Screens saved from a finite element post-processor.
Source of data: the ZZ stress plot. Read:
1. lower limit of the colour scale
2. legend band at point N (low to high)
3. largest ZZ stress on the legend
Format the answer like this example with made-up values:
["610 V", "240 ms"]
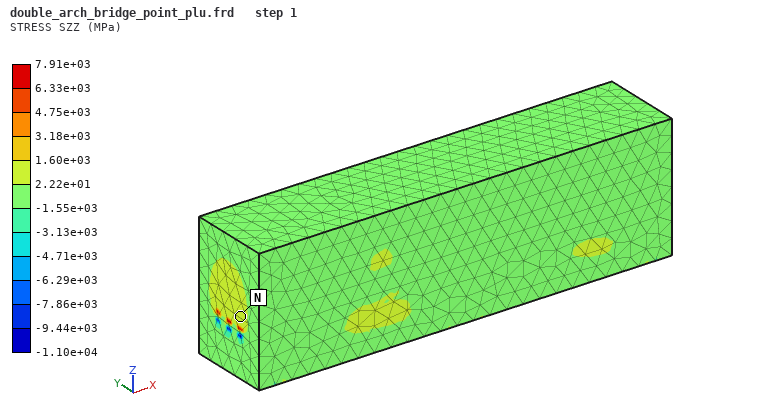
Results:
["-1.10e+04 MPa", "2.22e+01 to 1.60e+03 MPa", "7.91e+03 MPa"]
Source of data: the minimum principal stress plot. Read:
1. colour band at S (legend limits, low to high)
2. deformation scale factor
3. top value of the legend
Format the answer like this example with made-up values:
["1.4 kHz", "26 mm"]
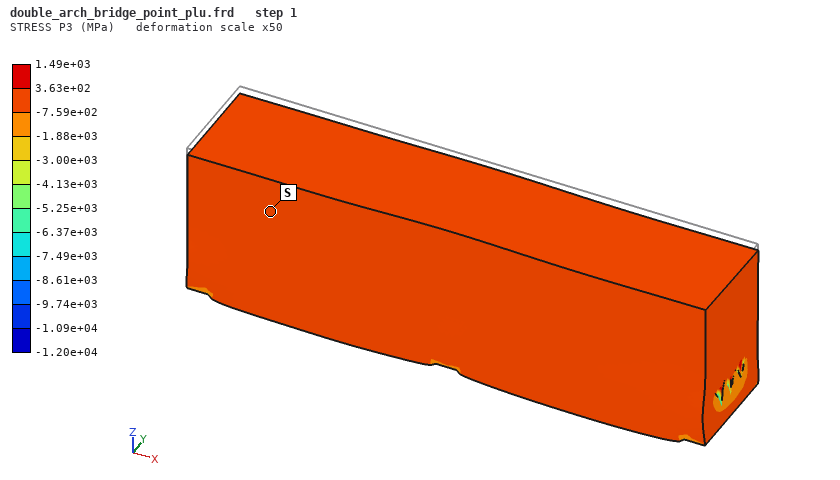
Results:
["-7.59e+02 to 3.63e+02 MPa", "50", "1.49e+03 MPa"]
